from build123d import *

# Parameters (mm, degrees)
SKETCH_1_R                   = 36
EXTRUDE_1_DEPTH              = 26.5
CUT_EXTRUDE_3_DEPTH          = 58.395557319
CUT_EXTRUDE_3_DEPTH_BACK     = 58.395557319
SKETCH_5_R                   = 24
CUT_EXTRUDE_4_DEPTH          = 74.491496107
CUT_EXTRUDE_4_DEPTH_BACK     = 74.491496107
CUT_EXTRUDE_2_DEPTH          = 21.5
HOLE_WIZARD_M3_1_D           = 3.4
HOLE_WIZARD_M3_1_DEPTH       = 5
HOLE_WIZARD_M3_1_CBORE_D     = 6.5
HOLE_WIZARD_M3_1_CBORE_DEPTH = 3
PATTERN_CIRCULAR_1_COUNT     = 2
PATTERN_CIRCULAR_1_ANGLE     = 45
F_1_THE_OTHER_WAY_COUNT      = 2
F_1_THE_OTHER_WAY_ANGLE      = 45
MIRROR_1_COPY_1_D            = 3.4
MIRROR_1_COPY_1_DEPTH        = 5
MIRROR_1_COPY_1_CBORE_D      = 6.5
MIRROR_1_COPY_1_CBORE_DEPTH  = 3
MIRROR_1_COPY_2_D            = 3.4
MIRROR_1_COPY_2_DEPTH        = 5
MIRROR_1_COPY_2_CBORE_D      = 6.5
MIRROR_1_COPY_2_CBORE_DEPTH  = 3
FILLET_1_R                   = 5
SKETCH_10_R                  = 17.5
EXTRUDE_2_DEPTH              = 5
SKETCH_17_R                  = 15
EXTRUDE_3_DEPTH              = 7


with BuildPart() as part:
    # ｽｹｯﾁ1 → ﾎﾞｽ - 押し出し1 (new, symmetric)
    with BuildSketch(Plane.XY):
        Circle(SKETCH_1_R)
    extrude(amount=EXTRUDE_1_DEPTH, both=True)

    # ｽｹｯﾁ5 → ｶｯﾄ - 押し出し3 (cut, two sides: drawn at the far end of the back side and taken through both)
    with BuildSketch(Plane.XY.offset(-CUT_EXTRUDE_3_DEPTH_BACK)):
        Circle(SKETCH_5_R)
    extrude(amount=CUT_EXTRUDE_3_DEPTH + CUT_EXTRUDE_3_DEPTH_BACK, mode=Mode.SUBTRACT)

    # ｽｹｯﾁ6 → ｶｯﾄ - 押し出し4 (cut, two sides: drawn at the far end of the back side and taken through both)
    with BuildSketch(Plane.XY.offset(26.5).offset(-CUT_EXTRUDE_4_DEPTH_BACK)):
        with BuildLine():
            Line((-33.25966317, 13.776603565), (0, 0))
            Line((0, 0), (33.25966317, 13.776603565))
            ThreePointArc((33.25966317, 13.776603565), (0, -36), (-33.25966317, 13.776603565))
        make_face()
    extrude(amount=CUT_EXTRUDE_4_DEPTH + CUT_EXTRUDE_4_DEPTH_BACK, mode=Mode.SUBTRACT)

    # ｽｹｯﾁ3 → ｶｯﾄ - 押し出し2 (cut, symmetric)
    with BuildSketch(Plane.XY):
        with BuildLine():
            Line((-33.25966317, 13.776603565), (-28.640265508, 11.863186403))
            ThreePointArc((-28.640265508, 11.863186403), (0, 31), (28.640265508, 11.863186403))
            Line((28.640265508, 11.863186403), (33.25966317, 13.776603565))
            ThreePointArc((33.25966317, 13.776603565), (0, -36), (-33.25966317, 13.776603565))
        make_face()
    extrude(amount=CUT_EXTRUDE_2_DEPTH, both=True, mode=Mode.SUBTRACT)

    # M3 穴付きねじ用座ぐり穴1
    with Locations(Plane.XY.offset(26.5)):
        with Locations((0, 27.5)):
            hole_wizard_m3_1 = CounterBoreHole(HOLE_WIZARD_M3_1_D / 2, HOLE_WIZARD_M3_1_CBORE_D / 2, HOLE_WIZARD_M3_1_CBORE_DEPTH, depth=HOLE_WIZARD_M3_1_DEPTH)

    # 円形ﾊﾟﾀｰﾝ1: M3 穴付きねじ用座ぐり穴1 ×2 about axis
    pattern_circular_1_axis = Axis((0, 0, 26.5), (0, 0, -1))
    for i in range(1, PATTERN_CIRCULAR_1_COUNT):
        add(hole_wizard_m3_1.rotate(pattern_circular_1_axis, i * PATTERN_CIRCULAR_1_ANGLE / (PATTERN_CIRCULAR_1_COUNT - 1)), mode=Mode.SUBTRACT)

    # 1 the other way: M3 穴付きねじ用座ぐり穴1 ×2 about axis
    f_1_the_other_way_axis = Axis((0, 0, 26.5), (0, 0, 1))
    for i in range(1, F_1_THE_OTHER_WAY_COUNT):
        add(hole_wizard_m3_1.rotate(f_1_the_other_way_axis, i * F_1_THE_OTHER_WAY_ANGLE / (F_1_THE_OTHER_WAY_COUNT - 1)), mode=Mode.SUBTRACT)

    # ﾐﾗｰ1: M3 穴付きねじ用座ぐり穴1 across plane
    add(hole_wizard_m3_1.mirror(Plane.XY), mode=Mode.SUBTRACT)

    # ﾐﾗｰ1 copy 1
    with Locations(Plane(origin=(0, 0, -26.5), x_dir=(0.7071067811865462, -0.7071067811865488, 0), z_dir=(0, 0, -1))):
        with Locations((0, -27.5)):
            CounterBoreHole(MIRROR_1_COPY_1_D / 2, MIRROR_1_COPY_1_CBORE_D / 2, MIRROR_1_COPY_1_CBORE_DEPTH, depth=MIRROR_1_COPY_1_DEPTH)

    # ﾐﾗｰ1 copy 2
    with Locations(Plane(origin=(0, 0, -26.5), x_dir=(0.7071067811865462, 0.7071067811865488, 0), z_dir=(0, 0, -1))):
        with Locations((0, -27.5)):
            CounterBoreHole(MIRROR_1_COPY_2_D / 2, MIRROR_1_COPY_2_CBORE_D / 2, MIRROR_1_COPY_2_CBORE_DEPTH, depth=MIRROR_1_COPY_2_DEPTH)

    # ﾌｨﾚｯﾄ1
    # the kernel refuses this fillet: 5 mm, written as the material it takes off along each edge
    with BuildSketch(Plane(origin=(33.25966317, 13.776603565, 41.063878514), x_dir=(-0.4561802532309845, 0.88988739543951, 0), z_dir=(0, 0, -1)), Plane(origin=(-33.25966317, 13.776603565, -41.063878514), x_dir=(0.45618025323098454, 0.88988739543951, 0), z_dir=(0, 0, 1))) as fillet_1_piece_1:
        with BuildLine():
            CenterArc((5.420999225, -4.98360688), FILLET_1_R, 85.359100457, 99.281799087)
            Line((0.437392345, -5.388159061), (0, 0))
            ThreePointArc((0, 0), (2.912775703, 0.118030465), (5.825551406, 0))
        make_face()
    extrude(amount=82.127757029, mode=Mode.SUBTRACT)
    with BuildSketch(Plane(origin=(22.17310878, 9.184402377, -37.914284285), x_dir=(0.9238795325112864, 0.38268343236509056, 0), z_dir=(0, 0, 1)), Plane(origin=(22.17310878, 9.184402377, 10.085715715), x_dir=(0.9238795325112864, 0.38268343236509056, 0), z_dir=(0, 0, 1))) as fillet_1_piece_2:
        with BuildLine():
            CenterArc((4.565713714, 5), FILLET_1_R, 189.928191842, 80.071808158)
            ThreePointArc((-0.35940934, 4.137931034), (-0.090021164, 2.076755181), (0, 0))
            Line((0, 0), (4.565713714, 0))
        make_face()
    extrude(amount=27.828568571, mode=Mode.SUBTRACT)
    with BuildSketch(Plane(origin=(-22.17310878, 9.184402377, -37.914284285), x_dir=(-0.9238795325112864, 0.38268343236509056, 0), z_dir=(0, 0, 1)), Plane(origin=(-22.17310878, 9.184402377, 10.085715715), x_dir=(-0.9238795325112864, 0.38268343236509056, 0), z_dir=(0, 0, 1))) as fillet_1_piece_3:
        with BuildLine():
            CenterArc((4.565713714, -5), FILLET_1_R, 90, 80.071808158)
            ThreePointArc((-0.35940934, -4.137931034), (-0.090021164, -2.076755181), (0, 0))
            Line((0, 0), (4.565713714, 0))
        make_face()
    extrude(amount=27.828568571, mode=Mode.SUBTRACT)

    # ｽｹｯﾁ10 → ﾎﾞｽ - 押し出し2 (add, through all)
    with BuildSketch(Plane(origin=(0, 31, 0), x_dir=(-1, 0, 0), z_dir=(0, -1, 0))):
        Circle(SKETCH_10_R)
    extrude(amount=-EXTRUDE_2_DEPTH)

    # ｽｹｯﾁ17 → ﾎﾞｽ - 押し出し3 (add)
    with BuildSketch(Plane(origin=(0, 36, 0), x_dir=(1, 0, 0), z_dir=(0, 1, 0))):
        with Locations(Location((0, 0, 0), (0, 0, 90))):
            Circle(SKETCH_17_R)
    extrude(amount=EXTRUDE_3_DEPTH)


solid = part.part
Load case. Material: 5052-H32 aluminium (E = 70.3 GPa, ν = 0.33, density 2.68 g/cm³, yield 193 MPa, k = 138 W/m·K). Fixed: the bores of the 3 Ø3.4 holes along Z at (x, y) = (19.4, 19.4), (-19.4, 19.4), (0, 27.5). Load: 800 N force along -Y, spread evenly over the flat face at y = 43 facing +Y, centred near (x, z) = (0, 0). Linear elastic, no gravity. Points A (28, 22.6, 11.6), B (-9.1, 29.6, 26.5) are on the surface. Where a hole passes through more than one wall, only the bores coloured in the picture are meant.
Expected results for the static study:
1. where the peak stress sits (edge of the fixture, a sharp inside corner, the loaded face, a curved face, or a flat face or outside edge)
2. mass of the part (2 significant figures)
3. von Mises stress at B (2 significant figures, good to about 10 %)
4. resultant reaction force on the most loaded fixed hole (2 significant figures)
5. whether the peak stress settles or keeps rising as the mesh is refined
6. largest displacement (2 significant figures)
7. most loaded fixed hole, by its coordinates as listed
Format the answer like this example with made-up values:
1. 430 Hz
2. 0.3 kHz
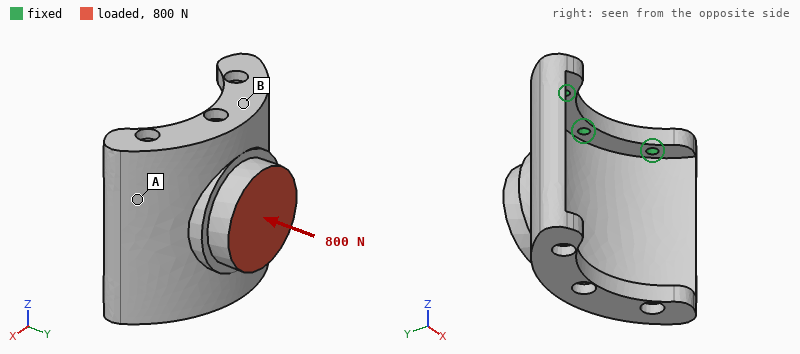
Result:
1. edge of the fixture
2. 80 g
3. 25 MPa
4. 1.5 kN
5. keeps rising
6. 0.17 mm
7. (0, 27.5)
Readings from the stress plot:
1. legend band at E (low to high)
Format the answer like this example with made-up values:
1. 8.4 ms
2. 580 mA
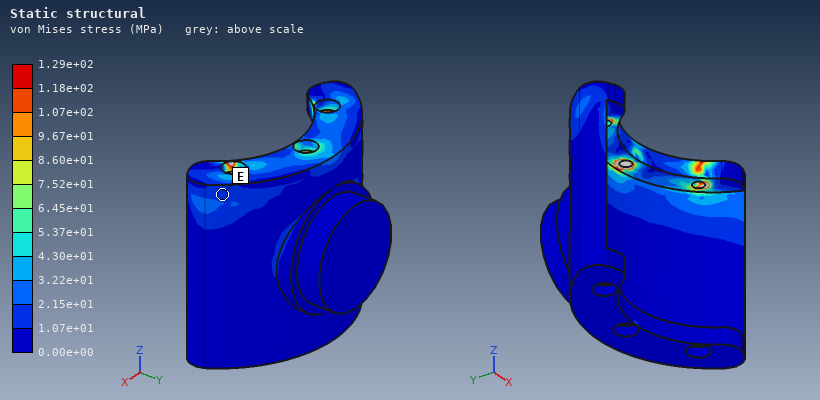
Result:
1. 1.07e+01 to 2.15e+01 MPa
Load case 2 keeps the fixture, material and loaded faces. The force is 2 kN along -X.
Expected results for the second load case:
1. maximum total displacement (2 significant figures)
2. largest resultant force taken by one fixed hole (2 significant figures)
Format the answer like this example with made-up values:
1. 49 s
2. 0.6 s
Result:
1. 50 µm
2. 1.4 kN
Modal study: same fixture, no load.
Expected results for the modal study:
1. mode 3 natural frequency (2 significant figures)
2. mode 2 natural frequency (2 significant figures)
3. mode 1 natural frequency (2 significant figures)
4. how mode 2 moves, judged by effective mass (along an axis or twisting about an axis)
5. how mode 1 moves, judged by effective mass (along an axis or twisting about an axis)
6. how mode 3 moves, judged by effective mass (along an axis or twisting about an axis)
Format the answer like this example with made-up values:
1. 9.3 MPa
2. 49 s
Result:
1. 5300 Hz
2. 2400 Hz
3. 1400 Hz
4. along X
5. along Y
6. along X
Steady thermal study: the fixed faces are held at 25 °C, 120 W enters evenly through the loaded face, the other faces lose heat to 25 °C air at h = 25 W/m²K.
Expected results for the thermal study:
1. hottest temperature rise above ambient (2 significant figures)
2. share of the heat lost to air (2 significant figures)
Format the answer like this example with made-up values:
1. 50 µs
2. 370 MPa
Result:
1. 85 K
2. 13 %
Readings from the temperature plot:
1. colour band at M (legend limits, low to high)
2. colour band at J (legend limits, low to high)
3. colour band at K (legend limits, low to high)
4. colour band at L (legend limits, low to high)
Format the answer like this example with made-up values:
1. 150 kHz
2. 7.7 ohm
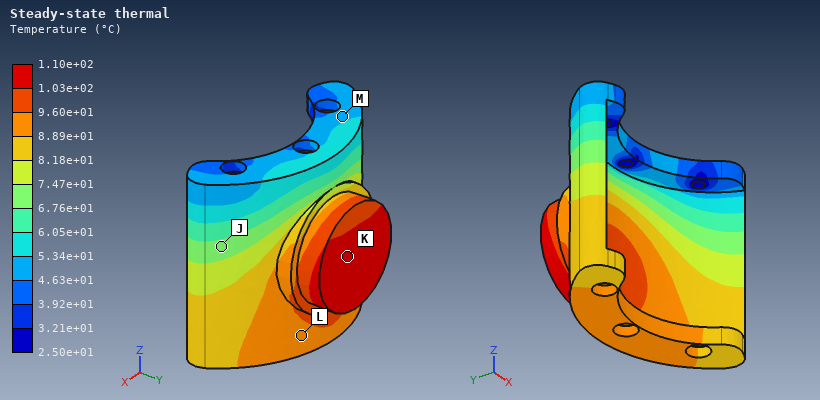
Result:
1. 4.63e+01 to 5.34e+01 °C
2. 6.76e+01 to 7.47e+01 °C
3. 1.03e+02 to 1.10e+02 °C
4. 8.89e+01 to 9.60e+01 °C
